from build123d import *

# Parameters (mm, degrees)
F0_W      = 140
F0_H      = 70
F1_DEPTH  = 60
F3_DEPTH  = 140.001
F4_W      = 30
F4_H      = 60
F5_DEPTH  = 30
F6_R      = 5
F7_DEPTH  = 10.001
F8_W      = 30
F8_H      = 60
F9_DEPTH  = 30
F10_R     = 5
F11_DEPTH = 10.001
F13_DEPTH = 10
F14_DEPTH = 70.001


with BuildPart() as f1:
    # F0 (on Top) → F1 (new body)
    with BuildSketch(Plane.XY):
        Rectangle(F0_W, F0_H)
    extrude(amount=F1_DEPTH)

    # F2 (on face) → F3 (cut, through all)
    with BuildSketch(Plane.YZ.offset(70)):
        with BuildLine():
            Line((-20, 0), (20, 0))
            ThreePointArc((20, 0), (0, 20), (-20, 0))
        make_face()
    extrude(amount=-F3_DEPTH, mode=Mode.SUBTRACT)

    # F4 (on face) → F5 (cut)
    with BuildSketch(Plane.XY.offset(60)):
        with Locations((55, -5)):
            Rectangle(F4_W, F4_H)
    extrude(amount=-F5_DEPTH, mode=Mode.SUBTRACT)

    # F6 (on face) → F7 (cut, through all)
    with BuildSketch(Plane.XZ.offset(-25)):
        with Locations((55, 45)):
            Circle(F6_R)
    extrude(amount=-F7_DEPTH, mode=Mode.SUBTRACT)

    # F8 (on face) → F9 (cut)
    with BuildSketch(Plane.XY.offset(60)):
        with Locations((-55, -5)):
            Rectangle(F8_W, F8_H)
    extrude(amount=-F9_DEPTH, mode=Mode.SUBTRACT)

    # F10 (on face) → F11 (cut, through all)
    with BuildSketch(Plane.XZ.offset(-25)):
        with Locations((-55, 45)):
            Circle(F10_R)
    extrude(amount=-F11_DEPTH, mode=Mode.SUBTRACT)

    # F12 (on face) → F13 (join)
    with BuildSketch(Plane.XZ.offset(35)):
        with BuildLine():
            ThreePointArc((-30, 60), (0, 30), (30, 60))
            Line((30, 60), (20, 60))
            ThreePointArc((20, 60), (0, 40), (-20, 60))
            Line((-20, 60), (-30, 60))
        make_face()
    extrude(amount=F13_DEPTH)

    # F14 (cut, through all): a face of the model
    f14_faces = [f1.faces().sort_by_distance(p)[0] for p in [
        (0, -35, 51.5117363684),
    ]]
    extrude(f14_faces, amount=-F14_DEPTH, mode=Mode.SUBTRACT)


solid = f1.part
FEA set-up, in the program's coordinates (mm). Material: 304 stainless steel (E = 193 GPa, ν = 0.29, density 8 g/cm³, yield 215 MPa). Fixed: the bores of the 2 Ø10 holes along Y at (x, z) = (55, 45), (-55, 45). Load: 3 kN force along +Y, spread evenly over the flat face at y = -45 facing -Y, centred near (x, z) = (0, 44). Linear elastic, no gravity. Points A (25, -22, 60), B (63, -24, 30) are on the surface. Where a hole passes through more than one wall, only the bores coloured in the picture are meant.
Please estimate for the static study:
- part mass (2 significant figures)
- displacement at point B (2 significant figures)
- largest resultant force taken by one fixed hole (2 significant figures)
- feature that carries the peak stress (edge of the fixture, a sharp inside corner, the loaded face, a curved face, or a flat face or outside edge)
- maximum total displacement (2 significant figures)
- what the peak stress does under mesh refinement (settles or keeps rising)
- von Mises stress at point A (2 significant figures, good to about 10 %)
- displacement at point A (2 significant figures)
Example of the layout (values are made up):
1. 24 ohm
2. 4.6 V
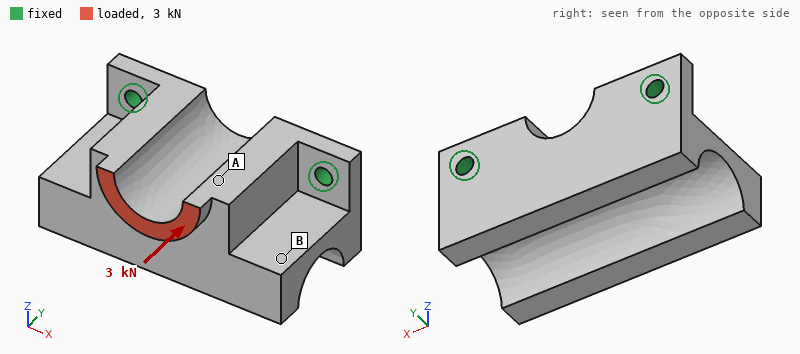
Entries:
1. 2.8 kg
2. 3.2 µm
3. 1.6 kN
4. edge of the fixture
5. 6.2 µm
6. keeps rising
7. 3.7 MPa
8. 4.6 µm
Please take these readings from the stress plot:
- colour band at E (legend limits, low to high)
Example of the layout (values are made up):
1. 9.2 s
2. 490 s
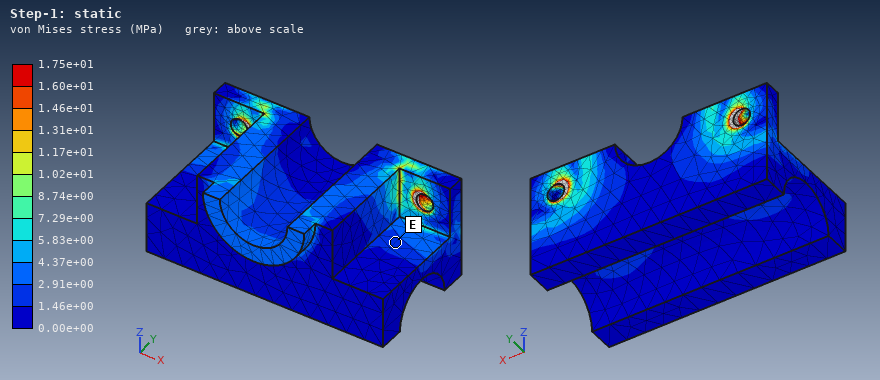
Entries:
1. 1.46e+00 to 2.91e+00 MPa
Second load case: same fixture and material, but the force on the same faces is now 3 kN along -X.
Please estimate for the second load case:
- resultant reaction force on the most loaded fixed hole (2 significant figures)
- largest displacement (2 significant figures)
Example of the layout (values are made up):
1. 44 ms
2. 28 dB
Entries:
1. 2.6 kN
2. 11 µm
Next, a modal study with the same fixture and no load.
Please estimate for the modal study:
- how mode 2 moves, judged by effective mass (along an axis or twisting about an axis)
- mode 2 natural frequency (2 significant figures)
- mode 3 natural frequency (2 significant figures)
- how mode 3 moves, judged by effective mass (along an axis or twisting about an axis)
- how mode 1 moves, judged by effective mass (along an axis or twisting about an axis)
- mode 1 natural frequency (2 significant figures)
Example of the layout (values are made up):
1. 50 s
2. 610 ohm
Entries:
1. along X
2. 3300 Hz
3. 3900 Hz
4. along X
5. along Z
6. 900 Hz
